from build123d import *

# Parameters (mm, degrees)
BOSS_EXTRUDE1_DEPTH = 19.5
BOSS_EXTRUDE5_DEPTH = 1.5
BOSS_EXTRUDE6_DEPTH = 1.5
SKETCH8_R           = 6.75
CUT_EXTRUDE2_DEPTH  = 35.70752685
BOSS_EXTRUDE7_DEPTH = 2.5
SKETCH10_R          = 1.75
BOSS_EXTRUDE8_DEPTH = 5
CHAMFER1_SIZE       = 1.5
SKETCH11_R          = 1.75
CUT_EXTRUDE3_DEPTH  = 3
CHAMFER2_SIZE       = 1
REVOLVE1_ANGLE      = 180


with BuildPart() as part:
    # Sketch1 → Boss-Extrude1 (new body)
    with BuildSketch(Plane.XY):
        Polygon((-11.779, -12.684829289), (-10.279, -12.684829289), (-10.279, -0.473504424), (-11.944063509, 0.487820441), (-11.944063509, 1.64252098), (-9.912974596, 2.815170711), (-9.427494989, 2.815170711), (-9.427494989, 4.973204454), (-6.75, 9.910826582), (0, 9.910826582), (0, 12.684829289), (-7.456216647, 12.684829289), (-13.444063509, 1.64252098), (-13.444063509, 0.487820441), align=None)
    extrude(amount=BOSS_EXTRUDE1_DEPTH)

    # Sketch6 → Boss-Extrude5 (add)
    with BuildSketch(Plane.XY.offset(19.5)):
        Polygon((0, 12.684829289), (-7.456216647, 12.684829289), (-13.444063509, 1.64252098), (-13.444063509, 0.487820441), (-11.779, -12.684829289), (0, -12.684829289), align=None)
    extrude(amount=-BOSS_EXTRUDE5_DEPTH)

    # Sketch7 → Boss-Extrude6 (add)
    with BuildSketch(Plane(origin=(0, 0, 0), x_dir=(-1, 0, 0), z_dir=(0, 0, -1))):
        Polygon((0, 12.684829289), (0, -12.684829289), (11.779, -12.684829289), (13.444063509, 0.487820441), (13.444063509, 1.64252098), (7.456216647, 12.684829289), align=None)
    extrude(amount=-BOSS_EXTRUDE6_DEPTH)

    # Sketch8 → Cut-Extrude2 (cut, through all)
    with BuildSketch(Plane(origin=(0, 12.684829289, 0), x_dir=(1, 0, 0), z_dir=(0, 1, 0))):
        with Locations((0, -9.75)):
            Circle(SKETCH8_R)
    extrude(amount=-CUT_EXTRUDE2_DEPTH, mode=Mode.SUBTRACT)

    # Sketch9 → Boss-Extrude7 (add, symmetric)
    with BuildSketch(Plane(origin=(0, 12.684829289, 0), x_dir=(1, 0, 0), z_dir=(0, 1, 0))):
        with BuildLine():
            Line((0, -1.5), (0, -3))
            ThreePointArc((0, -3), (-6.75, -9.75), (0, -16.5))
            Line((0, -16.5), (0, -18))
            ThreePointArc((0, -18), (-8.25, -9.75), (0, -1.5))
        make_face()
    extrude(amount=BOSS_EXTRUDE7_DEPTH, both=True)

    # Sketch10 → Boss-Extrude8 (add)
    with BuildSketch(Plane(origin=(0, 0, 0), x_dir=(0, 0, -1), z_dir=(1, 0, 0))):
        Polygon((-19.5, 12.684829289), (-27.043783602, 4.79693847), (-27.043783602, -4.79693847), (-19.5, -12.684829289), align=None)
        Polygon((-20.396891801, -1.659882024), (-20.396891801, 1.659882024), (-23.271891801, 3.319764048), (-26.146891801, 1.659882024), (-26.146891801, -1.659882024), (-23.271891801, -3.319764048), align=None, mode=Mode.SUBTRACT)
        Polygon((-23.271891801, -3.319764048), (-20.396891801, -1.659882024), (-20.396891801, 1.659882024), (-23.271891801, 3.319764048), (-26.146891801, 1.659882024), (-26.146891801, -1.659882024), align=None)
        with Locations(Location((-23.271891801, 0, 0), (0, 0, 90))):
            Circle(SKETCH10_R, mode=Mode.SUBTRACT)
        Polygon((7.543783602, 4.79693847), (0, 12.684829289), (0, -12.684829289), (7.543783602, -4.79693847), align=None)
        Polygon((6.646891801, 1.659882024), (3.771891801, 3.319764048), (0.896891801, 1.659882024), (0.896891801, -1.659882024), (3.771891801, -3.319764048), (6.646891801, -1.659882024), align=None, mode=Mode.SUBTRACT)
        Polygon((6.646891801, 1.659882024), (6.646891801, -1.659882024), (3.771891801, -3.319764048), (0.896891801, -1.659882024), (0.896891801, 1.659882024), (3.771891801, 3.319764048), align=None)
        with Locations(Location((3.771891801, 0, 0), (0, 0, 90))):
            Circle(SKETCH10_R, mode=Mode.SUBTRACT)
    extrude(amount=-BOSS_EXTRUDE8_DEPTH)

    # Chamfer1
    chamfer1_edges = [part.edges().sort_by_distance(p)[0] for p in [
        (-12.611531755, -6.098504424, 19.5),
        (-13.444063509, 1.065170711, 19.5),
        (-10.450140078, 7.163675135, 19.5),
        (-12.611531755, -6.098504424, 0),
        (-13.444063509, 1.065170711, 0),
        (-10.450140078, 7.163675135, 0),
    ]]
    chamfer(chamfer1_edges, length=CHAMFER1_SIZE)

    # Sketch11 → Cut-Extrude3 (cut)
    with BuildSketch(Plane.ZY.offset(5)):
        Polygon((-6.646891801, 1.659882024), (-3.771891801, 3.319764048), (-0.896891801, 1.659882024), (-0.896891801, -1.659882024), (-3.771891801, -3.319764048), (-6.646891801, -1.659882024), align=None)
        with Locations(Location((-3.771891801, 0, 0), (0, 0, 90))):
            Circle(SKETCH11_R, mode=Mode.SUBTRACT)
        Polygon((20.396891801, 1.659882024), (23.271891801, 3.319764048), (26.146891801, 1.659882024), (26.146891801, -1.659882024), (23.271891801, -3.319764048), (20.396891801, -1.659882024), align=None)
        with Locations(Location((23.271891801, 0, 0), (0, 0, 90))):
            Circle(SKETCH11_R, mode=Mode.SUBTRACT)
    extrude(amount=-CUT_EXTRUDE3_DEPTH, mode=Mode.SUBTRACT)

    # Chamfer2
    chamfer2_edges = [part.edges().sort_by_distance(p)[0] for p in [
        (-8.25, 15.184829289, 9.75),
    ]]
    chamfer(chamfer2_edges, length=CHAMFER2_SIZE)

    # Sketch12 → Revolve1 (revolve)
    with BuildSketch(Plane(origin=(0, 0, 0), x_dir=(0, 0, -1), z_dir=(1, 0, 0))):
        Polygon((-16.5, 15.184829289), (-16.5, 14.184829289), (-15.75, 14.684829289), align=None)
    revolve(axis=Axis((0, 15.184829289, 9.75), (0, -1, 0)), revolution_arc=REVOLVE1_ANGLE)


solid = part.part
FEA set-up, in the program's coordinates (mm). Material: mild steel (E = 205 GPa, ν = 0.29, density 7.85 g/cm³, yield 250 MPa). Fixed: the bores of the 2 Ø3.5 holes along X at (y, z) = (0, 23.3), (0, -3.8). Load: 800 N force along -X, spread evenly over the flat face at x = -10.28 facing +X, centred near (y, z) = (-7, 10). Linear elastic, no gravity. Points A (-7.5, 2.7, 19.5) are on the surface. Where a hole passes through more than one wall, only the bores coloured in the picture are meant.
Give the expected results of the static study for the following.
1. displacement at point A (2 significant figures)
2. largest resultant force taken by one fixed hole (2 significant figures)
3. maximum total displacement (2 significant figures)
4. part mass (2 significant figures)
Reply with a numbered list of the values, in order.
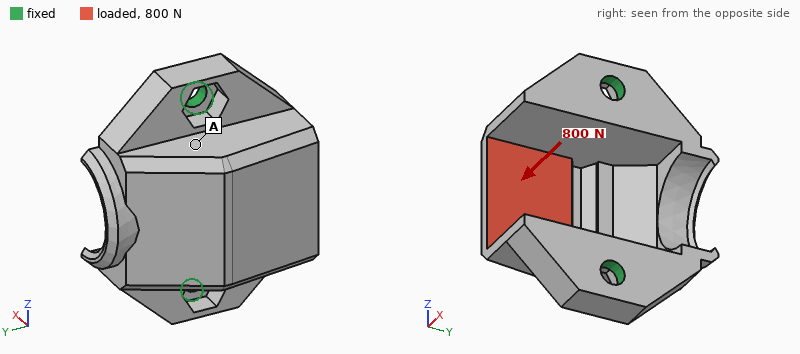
1. 7.4 µm
2. 450 N
3. 36 µm
4. 24 g
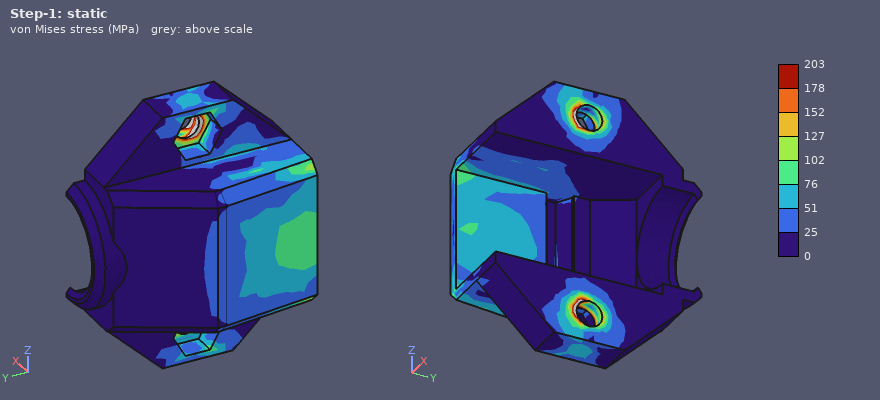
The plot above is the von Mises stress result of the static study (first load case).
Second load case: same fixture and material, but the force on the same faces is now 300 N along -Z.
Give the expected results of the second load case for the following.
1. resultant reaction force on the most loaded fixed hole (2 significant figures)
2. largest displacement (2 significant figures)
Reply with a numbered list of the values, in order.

1. 170 N
2. 11 µm
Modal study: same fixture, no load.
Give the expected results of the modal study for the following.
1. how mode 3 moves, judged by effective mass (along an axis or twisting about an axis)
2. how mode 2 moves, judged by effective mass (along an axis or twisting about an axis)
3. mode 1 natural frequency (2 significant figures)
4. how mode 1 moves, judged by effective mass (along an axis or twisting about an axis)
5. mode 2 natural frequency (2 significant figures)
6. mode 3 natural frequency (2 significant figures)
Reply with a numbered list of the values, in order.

1. along Z
2. along Z
3. 7200 Hz
4. along Y
5. 12 kHz
6. 16 kHz
